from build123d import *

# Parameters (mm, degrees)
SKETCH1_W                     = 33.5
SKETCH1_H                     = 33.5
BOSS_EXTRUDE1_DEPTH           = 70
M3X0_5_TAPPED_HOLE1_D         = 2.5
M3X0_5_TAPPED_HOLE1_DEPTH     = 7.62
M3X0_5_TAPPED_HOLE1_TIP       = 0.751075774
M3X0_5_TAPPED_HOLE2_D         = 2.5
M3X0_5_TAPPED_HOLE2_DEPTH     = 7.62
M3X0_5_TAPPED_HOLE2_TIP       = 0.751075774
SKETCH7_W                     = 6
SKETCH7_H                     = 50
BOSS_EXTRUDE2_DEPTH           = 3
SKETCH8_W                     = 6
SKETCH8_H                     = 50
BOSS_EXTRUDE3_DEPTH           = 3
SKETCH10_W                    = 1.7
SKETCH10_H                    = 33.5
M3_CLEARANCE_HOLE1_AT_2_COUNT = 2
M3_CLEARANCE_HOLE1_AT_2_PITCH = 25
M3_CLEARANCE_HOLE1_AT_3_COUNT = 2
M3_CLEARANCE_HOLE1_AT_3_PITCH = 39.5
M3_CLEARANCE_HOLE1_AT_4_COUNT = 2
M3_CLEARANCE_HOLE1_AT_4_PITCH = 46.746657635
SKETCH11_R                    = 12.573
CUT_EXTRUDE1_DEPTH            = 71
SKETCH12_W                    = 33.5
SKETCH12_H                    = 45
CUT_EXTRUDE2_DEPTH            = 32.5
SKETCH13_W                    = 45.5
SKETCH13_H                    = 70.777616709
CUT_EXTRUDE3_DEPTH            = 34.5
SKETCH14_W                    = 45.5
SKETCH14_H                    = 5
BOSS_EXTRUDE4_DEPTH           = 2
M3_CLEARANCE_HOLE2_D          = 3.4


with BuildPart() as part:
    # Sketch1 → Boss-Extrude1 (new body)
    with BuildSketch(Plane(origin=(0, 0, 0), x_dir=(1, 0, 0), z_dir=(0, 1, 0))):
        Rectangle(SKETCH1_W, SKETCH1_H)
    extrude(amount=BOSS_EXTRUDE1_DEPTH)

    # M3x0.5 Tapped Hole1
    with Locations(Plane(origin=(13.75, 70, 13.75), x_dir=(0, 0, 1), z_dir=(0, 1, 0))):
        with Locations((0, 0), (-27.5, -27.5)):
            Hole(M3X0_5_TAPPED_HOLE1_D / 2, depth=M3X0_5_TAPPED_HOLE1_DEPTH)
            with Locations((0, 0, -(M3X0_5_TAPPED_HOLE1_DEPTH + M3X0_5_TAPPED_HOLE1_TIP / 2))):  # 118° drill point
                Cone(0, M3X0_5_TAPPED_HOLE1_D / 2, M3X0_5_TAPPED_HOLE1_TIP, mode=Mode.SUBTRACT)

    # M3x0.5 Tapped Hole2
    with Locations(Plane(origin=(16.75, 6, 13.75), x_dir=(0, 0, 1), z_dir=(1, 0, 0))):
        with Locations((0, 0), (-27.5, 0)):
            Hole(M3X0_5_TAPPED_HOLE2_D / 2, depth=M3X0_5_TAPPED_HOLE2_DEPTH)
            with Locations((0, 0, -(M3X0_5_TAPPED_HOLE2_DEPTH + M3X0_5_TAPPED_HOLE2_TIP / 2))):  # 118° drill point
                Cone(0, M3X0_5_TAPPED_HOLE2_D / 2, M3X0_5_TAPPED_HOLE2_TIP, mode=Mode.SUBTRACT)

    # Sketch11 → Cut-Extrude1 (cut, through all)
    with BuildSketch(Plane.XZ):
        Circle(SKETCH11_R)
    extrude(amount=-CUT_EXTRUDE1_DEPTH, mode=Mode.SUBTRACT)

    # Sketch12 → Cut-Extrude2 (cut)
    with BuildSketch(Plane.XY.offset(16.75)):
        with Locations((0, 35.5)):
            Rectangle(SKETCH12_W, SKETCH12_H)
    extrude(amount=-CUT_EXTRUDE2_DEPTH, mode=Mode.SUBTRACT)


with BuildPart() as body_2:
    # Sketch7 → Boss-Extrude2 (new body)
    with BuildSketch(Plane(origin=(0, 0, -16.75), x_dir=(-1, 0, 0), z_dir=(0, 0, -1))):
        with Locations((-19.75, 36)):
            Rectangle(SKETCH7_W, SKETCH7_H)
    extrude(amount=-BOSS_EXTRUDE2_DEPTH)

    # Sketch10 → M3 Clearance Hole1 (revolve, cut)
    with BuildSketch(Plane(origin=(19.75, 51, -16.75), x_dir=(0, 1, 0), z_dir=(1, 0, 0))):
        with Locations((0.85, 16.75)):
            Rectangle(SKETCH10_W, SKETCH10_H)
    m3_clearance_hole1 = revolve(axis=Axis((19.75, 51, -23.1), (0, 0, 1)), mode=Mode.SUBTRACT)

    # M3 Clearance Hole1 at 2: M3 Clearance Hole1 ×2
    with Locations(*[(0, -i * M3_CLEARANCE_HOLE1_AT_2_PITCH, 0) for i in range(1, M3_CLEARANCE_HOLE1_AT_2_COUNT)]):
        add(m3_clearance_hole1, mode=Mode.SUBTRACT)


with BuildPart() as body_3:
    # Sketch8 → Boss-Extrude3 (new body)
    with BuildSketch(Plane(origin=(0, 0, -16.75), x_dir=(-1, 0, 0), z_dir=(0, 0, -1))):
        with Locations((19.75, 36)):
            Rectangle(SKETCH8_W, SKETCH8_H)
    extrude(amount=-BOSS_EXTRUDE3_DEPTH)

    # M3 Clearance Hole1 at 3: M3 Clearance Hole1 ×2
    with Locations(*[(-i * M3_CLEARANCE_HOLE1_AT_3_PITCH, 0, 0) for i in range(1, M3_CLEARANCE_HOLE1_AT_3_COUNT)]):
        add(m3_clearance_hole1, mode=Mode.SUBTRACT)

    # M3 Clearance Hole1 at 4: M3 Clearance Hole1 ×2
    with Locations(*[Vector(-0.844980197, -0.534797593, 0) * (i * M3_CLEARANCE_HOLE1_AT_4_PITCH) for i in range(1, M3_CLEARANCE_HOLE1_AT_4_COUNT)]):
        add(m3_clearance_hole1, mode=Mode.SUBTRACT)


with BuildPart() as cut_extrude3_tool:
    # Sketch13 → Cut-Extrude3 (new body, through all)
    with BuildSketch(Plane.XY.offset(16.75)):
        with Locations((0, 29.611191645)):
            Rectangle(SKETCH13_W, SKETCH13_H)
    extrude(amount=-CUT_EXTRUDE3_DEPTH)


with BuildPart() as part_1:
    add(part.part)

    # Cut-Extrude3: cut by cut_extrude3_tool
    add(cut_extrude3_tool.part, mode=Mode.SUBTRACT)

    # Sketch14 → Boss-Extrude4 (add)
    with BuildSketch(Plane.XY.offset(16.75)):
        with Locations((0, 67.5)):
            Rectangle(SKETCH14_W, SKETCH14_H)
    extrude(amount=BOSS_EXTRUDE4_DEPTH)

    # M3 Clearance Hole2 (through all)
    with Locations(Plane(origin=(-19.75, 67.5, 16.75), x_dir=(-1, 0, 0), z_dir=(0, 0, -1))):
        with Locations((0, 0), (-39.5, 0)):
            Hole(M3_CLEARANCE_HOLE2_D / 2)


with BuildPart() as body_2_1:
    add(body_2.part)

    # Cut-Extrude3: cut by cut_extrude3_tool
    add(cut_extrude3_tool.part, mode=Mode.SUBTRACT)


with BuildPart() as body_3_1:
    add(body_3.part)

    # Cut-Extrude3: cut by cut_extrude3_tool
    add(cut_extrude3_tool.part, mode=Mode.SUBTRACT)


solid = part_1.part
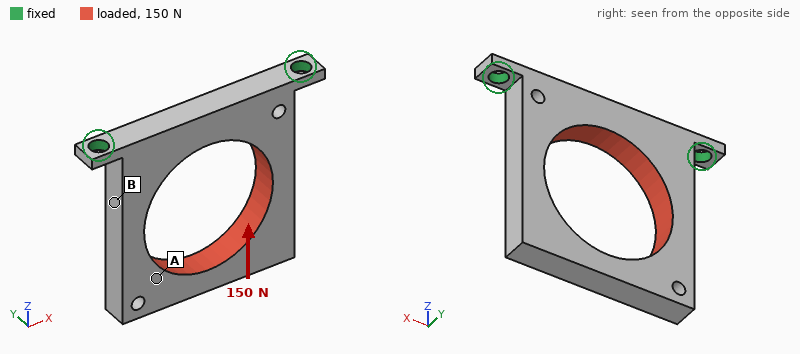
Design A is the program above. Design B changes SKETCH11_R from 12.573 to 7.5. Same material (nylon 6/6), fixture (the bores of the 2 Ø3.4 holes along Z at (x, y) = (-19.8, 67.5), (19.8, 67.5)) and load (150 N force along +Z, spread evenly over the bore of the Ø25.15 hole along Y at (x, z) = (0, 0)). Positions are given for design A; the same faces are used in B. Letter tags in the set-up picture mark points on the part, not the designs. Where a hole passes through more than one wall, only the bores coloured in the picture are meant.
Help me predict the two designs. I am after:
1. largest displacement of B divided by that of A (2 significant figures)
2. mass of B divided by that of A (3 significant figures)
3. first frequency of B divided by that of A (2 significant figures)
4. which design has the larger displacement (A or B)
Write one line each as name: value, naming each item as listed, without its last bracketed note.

largest displacement of B divided by that of A: 0.73
mass of B divided by that of A: 1.46
first frequency of B divided by that of A: 0.87
which design has the larger displacement: A
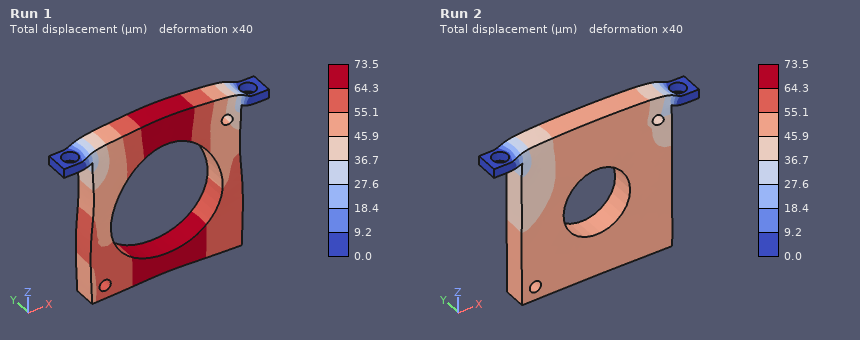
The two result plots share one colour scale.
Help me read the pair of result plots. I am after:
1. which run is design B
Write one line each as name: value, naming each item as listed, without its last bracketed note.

which run is design B: Run 2
